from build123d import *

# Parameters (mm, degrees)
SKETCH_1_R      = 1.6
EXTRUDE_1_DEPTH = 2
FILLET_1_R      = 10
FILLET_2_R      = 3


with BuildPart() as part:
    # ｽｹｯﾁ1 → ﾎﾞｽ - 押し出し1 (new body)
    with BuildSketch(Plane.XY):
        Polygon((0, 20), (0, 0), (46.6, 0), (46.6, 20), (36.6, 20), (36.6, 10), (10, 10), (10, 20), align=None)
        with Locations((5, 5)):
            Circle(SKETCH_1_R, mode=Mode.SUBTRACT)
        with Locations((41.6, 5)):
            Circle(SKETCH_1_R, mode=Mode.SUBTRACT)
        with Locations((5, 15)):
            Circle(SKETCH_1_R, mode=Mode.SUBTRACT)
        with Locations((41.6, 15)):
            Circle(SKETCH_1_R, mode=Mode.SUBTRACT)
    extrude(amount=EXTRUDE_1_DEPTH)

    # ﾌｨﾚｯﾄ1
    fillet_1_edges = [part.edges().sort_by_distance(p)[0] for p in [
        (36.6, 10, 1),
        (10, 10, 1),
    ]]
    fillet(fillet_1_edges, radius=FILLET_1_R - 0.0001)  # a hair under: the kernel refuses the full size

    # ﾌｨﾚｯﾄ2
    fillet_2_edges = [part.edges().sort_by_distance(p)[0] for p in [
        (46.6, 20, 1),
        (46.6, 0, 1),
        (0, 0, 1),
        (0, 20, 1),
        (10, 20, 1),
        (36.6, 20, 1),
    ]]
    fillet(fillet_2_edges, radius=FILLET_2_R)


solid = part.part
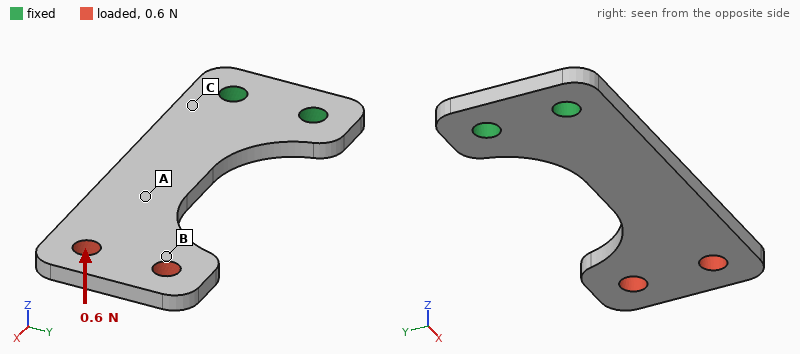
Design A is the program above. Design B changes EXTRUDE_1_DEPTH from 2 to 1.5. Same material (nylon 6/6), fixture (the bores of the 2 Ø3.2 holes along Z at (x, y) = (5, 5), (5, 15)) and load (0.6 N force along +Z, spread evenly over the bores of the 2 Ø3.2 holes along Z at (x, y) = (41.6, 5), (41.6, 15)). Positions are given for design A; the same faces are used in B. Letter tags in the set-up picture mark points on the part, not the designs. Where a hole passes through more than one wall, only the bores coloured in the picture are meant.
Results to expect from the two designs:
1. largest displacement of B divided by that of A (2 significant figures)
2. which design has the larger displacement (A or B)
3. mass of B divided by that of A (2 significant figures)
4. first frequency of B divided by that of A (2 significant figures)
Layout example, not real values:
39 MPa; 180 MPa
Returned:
2.3; B; 0.75; 0.76
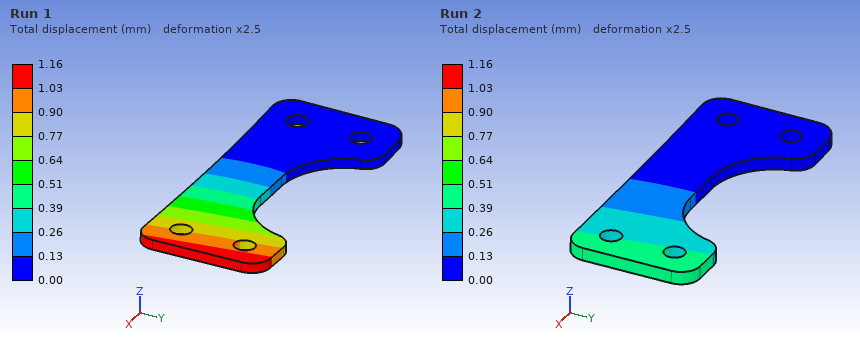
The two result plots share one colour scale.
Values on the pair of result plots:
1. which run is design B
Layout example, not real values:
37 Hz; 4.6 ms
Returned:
Run 1
